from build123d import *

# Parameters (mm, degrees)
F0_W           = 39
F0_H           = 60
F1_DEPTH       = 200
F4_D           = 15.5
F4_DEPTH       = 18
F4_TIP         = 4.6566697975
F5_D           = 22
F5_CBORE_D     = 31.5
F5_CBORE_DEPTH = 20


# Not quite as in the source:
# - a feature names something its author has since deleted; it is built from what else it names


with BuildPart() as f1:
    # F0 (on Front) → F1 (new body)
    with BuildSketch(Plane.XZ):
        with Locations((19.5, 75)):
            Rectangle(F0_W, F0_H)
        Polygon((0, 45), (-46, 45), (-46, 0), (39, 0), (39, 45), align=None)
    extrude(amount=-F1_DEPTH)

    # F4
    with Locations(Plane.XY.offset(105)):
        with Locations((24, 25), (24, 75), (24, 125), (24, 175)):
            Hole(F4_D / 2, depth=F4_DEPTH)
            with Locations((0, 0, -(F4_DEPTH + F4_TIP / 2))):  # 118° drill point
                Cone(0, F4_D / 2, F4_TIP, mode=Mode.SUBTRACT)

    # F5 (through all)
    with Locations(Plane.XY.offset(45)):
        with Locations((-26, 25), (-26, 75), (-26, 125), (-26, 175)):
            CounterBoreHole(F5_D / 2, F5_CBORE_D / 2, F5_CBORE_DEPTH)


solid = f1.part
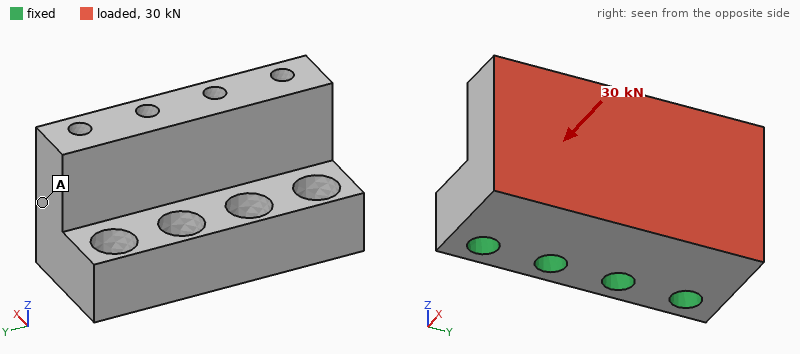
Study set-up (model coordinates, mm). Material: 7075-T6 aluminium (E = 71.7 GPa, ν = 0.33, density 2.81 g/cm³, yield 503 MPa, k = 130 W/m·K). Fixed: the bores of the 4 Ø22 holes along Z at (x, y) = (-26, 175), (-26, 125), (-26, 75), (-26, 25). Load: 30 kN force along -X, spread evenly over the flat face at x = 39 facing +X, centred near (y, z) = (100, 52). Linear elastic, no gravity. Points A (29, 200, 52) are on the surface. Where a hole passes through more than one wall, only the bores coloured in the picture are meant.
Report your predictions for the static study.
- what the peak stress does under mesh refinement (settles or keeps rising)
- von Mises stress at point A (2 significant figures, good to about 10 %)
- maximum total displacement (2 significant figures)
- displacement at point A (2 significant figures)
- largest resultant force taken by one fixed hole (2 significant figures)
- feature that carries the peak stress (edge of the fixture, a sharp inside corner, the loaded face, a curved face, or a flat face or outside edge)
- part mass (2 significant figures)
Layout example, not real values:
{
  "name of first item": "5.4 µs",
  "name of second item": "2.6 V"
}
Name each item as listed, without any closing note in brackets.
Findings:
{
  "what the peak stress does under mesh refinement": "keeps rising",
  "von Mises stress at point A": "5.8 MPa",
  "maximum total displacement": "93 µm",
  "displacement at point A": "44 µm",
  "largest resultant force taken by one fixed hole": "7.8 kN",
  "feature that carries the peak stress": "edge of the fixture",
  "part mass": "3.1 kg"
}
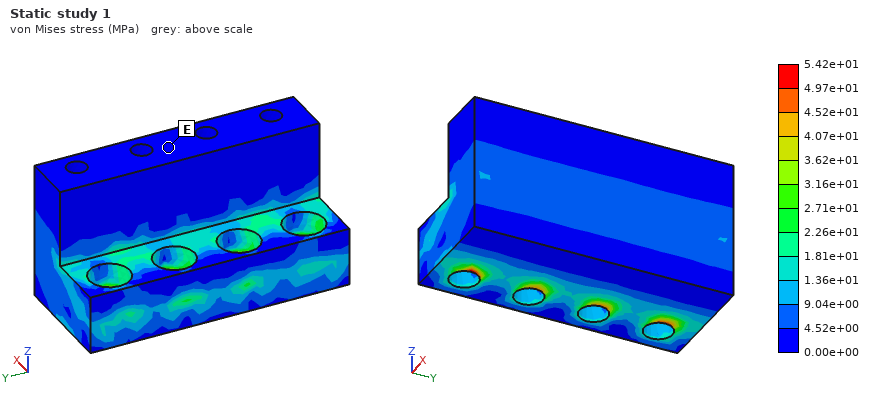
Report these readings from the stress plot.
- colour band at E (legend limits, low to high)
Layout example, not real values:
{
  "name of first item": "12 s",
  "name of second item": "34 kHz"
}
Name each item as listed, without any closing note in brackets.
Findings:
{
  "colour band at E": "0.00e+00 to 4.52e+00 MPa"
}
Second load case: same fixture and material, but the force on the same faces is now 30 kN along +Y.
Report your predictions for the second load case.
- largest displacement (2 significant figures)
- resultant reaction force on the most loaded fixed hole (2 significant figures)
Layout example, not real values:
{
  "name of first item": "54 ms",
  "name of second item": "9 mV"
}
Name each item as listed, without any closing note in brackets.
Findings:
{
  "largest displacement": "23 µm",
  "resultant reaction force on the most loaded fixed hole": "14 kN"
}
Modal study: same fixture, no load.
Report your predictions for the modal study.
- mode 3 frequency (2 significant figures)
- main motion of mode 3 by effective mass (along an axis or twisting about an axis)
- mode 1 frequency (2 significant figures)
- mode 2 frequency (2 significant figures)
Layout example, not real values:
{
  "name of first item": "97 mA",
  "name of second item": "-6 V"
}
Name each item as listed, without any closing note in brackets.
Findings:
{
  "mode 3 frequency": "5300 Hz",
  "main motion of mode 3 by effective mass": "along Y",
  "mode 1 frequency": "2100 Hz",
  "mode 2 frequency": "3300 Hz"
}
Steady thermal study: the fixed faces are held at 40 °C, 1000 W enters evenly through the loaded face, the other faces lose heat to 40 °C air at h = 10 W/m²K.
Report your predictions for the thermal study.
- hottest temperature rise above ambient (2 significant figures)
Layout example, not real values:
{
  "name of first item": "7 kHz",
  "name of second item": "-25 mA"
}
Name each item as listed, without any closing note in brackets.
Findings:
{
  "hottest temperature rise above ambient": "68 K"
}
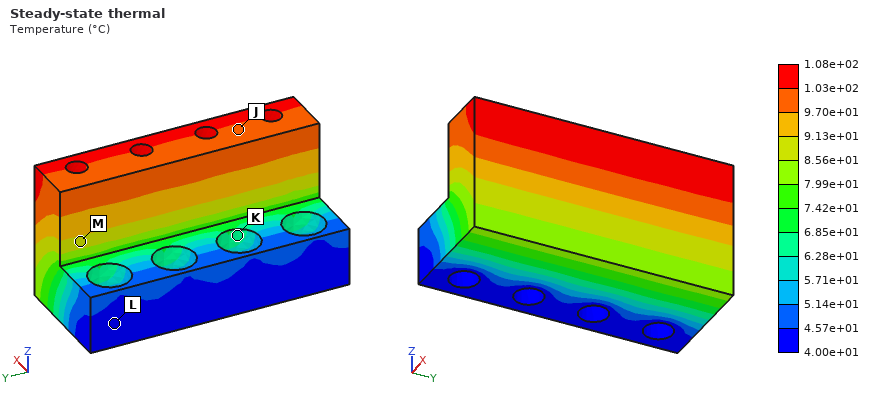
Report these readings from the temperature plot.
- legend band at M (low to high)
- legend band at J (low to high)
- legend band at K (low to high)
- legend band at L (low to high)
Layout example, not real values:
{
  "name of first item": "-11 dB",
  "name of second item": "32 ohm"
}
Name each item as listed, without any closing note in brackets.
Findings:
{
  "legend band at M": "8.56e+01 to 9.13e+01 °C",
  "legend band at J": "9.70e+01 to 1.03e+02 °C",
  "legend band at K": "6.28e+01 to 6.85e+01 °C",
  "legend band at L": "4.00e+01 to 4.57e+01 °C"
}
